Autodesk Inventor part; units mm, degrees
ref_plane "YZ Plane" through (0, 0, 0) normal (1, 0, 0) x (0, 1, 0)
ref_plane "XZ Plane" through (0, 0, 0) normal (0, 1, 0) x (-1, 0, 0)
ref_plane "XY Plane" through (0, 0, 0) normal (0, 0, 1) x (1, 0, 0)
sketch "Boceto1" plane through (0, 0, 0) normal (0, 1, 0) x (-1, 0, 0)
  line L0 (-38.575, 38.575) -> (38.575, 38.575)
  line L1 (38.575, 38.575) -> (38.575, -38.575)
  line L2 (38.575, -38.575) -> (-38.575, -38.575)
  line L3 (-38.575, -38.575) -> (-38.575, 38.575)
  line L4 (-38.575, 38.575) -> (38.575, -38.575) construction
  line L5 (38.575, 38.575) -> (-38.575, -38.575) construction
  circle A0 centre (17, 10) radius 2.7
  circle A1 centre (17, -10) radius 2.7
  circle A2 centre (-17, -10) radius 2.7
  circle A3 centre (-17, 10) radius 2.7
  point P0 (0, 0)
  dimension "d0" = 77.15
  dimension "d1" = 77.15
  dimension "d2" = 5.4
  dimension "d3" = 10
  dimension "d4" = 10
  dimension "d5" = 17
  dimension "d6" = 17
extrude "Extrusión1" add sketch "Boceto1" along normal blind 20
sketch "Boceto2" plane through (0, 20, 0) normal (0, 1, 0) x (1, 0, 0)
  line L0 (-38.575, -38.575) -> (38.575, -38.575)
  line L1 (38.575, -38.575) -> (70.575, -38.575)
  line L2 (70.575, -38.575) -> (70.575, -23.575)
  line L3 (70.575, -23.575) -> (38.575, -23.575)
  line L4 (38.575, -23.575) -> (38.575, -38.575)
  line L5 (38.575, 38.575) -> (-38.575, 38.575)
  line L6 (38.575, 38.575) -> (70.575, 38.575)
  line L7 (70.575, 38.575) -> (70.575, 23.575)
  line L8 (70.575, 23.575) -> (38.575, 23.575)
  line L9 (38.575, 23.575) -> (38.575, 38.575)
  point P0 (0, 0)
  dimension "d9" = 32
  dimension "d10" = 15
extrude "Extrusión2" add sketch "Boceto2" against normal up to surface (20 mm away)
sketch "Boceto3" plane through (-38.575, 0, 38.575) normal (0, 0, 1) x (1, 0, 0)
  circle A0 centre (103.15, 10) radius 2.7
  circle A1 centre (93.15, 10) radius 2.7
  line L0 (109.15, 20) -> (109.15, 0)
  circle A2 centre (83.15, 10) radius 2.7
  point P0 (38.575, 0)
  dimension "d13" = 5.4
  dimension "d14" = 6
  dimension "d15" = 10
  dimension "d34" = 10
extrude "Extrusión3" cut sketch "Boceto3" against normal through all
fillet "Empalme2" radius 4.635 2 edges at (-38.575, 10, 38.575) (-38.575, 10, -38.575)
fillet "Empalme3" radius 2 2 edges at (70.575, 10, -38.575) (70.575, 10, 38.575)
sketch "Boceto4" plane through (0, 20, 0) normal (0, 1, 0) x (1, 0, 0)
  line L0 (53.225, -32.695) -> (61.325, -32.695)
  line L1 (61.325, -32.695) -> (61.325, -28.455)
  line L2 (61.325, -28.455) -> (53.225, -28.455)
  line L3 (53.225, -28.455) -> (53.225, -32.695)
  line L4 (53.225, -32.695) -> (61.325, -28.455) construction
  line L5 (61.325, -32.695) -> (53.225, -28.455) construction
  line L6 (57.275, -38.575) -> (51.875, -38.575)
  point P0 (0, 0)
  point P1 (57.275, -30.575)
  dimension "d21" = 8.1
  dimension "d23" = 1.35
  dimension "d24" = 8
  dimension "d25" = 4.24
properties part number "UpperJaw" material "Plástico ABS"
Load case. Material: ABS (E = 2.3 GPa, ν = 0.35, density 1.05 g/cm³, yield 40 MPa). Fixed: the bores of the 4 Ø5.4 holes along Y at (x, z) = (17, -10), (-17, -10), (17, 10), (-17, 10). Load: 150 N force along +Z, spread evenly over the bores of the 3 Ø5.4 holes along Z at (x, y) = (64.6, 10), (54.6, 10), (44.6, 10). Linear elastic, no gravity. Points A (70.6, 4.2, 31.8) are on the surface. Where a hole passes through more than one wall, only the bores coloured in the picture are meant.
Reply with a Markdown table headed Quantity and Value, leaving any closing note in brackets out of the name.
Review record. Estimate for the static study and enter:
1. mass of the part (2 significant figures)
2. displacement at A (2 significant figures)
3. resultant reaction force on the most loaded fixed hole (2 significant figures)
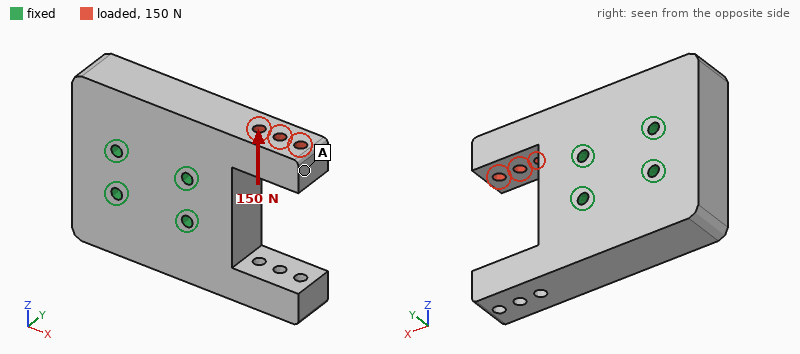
| Quantity | Value |
|---|---|
| mass of the part | 140 g |
| displacement at A | 0.16 mm |
| resultant reaction force on the most loaded fixed hole | 140 N |
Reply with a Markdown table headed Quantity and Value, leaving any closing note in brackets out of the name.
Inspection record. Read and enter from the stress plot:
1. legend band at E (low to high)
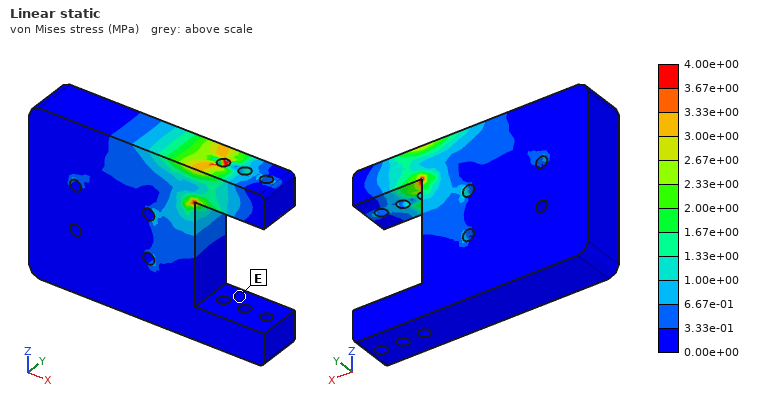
| Quantity | Value |
|---|---|
| legend band at E | 0.00e+00 to 3.33e-01 MPa |
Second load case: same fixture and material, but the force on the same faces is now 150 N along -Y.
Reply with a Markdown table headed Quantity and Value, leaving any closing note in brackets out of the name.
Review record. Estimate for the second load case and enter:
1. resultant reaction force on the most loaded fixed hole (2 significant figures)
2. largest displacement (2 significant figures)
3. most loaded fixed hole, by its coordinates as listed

| Quantity | Value |
|---|---|
| resultant reaction force on the most loaded fixed hole | 220 N |
| largest displacement | 0.22 mm |
| most loaded fixed hole, by its coordinates as listed | (17, 10) |
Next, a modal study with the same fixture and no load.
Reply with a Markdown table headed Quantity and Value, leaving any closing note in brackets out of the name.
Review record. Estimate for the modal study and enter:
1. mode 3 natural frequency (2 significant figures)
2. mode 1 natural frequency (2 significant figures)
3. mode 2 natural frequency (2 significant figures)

| Quantity | Value |
|---|---|
| mode 3 natural frequency | 1900 Hz |
| mode 1 natural frequency | 1600 Hz |
| mode 2 natural frequency | 1600 Hz |
